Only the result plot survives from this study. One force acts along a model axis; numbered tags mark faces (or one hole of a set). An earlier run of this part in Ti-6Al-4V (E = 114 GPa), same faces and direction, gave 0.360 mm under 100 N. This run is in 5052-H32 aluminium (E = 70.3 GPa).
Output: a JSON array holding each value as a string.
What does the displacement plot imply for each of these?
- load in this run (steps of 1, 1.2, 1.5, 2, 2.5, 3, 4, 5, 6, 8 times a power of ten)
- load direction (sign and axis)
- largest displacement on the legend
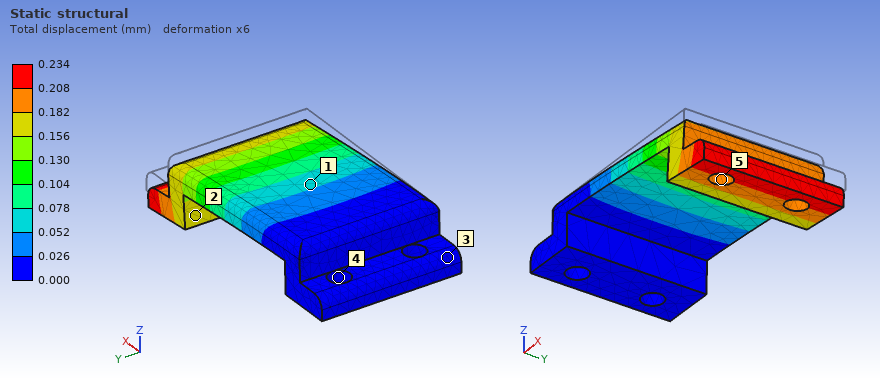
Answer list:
["40 N", "-Z", "0.234 mm"]
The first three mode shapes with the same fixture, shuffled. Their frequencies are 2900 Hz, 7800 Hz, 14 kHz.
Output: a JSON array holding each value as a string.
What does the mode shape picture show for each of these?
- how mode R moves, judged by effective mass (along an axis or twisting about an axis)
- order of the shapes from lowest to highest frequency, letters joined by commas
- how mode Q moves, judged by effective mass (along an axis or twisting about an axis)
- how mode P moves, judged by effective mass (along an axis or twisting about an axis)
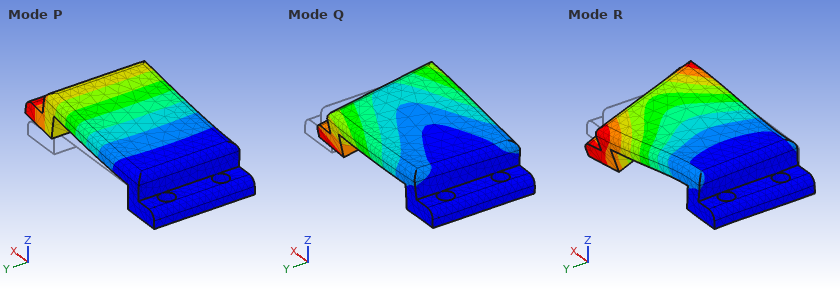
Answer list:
["along Y", "P, Q, R", "along Y", "along Z"]
